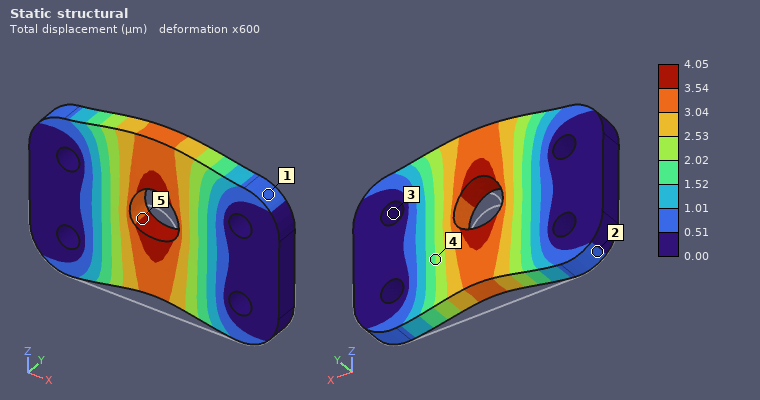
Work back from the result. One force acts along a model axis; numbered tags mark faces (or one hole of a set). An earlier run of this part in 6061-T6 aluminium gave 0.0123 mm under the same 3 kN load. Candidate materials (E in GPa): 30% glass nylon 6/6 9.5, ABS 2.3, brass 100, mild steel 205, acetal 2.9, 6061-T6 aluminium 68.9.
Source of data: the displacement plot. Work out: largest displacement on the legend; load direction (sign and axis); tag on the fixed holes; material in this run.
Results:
4.05 µm
+Z
3
mild steel
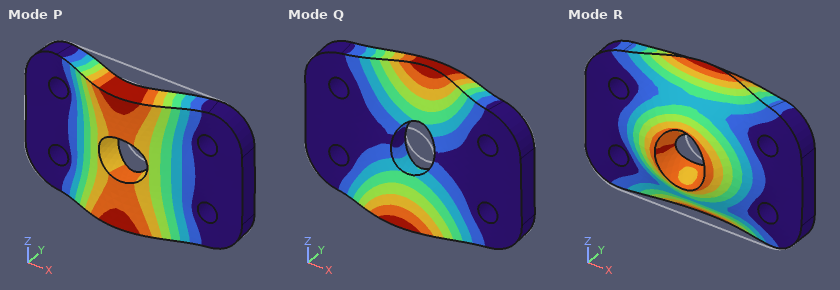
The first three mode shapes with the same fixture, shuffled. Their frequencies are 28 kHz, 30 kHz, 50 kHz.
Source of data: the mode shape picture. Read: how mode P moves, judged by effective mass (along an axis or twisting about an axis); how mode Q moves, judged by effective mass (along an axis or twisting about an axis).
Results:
along Y
twisting about X
